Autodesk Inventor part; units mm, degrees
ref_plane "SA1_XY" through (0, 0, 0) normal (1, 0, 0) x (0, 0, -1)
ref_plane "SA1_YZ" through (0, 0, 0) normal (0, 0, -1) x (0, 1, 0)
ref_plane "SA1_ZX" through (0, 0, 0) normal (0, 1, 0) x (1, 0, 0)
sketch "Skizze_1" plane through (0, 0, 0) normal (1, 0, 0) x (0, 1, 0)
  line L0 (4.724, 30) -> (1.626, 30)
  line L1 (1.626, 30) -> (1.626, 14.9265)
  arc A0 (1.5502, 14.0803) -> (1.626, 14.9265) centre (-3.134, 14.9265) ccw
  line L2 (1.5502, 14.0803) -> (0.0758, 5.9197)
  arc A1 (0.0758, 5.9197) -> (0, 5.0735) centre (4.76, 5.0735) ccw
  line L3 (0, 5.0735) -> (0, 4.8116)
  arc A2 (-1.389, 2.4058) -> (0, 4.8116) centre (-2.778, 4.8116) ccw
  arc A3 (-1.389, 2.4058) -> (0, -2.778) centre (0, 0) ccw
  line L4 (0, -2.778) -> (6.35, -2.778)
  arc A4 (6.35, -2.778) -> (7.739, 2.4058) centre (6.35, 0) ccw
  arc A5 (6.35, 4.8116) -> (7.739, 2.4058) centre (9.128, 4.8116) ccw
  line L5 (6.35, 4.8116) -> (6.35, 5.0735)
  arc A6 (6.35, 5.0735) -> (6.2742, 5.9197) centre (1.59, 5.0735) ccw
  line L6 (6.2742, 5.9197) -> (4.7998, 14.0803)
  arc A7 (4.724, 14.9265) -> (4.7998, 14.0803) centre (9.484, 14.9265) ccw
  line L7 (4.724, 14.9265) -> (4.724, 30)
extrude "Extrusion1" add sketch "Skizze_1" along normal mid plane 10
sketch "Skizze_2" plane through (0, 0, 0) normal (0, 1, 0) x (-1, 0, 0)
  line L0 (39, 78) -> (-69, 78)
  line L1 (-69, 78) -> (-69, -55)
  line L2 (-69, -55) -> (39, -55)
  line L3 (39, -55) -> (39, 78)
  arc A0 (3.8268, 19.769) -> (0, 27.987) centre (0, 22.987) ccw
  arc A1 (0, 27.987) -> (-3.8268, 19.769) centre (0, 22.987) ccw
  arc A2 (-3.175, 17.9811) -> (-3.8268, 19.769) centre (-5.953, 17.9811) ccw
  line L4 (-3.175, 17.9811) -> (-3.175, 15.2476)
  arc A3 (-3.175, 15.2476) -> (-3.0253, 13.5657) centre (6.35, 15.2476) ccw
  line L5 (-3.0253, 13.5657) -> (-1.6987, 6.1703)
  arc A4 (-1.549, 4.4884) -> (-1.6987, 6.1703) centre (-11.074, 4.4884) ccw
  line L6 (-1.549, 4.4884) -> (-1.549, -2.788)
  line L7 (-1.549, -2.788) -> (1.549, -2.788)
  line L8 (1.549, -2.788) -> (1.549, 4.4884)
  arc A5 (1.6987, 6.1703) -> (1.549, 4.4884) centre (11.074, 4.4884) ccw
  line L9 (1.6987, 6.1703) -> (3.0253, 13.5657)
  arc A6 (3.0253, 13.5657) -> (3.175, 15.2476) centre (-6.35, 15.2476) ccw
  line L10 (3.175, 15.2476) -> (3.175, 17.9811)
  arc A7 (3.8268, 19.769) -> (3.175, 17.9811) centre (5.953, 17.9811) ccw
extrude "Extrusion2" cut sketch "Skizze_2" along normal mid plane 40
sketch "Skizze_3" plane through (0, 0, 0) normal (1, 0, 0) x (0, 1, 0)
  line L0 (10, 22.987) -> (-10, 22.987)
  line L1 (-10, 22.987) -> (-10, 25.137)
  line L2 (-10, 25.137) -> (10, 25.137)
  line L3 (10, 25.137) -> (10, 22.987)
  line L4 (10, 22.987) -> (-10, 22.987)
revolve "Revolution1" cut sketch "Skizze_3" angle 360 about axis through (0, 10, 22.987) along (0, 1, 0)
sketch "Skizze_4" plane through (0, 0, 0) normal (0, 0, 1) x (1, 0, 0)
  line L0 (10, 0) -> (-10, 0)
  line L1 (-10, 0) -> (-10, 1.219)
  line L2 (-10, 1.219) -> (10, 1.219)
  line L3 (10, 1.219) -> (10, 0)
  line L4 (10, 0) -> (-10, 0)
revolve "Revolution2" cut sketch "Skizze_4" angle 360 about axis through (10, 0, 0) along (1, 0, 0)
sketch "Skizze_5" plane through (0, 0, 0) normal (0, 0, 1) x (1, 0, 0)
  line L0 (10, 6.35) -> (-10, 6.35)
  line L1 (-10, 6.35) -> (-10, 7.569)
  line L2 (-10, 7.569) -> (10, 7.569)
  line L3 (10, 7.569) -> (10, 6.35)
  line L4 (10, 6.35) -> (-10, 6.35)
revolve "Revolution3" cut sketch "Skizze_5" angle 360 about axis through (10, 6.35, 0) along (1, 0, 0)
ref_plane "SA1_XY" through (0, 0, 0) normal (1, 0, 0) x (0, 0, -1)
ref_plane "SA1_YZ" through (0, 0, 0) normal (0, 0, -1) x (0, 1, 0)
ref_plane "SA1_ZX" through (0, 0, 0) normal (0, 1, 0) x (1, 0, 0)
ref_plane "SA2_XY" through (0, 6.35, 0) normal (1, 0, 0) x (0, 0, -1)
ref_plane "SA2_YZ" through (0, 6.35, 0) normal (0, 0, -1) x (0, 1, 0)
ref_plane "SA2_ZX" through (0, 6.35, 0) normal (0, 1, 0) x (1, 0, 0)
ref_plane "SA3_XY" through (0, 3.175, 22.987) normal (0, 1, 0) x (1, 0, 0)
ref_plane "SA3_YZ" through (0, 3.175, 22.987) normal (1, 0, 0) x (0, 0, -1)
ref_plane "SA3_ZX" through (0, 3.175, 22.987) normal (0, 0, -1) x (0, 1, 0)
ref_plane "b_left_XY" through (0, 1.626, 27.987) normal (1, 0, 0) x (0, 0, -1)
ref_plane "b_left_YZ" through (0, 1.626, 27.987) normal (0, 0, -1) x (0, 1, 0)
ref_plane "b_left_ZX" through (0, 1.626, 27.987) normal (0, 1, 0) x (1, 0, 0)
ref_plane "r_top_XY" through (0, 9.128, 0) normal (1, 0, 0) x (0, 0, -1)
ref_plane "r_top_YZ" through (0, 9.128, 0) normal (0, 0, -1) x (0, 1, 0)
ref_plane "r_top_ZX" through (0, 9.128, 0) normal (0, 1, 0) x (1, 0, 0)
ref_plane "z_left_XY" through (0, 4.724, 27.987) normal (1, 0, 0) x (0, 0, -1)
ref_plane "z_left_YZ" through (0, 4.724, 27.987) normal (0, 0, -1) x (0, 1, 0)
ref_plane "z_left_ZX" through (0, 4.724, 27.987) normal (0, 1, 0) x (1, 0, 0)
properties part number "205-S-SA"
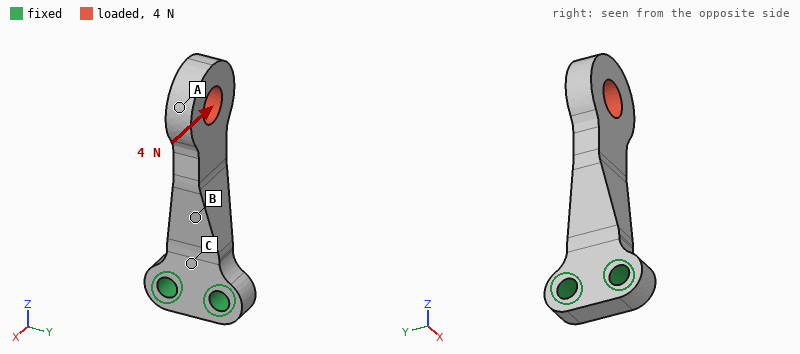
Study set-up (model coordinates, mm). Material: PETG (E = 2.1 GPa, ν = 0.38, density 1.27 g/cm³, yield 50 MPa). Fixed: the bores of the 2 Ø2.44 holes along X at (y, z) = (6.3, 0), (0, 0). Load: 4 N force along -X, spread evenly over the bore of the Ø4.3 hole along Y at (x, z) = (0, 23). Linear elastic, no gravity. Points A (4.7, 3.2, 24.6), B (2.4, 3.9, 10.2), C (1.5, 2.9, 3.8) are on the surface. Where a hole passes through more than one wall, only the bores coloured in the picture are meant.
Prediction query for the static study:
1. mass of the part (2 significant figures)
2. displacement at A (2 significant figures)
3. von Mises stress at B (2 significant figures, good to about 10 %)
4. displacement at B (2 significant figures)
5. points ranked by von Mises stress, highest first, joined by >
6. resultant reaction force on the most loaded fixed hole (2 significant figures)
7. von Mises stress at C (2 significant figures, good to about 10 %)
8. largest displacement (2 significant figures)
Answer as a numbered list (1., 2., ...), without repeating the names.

1. 0.87 g
2. 0.36 mm
3. 2.9 MPa
4. 0.097 mm
5. C > B > A
6. 2.0 N
7. 6.3 MPa
8. 0.41 mm
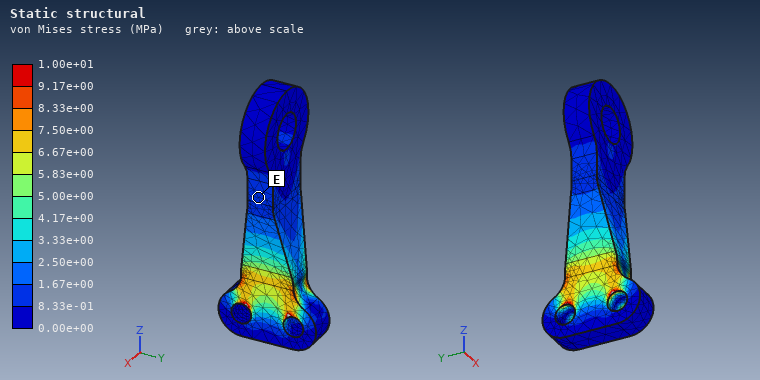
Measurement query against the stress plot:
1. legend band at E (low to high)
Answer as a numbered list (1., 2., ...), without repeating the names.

1. 8.33e-01 to 1.67e+00 MPa
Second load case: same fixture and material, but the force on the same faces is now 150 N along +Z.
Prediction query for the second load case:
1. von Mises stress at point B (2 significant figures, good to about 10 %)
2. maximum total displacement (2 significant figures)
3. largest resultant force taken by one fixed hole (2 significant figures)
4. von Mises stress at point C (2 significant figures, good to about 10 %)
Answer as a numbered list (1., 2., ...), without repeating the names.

1. 6.9 MPa
2. 0.10 mm
3. 80 N
4. 6.0 MPa
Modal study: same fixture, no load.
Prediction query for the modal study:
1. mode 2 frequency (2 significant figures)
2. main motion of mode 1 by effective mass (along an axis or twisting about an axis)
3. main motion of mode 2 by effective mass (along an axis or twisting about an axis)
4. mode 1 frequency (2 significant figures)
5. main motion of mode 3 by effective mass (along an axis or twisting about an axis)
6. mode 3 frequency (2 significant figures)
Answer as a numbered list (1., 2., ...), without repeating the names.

1. 1600 Hz
2. along X
3. along Y
4. 990 Hz
5. twisting about Z
6. 4700 Hz
